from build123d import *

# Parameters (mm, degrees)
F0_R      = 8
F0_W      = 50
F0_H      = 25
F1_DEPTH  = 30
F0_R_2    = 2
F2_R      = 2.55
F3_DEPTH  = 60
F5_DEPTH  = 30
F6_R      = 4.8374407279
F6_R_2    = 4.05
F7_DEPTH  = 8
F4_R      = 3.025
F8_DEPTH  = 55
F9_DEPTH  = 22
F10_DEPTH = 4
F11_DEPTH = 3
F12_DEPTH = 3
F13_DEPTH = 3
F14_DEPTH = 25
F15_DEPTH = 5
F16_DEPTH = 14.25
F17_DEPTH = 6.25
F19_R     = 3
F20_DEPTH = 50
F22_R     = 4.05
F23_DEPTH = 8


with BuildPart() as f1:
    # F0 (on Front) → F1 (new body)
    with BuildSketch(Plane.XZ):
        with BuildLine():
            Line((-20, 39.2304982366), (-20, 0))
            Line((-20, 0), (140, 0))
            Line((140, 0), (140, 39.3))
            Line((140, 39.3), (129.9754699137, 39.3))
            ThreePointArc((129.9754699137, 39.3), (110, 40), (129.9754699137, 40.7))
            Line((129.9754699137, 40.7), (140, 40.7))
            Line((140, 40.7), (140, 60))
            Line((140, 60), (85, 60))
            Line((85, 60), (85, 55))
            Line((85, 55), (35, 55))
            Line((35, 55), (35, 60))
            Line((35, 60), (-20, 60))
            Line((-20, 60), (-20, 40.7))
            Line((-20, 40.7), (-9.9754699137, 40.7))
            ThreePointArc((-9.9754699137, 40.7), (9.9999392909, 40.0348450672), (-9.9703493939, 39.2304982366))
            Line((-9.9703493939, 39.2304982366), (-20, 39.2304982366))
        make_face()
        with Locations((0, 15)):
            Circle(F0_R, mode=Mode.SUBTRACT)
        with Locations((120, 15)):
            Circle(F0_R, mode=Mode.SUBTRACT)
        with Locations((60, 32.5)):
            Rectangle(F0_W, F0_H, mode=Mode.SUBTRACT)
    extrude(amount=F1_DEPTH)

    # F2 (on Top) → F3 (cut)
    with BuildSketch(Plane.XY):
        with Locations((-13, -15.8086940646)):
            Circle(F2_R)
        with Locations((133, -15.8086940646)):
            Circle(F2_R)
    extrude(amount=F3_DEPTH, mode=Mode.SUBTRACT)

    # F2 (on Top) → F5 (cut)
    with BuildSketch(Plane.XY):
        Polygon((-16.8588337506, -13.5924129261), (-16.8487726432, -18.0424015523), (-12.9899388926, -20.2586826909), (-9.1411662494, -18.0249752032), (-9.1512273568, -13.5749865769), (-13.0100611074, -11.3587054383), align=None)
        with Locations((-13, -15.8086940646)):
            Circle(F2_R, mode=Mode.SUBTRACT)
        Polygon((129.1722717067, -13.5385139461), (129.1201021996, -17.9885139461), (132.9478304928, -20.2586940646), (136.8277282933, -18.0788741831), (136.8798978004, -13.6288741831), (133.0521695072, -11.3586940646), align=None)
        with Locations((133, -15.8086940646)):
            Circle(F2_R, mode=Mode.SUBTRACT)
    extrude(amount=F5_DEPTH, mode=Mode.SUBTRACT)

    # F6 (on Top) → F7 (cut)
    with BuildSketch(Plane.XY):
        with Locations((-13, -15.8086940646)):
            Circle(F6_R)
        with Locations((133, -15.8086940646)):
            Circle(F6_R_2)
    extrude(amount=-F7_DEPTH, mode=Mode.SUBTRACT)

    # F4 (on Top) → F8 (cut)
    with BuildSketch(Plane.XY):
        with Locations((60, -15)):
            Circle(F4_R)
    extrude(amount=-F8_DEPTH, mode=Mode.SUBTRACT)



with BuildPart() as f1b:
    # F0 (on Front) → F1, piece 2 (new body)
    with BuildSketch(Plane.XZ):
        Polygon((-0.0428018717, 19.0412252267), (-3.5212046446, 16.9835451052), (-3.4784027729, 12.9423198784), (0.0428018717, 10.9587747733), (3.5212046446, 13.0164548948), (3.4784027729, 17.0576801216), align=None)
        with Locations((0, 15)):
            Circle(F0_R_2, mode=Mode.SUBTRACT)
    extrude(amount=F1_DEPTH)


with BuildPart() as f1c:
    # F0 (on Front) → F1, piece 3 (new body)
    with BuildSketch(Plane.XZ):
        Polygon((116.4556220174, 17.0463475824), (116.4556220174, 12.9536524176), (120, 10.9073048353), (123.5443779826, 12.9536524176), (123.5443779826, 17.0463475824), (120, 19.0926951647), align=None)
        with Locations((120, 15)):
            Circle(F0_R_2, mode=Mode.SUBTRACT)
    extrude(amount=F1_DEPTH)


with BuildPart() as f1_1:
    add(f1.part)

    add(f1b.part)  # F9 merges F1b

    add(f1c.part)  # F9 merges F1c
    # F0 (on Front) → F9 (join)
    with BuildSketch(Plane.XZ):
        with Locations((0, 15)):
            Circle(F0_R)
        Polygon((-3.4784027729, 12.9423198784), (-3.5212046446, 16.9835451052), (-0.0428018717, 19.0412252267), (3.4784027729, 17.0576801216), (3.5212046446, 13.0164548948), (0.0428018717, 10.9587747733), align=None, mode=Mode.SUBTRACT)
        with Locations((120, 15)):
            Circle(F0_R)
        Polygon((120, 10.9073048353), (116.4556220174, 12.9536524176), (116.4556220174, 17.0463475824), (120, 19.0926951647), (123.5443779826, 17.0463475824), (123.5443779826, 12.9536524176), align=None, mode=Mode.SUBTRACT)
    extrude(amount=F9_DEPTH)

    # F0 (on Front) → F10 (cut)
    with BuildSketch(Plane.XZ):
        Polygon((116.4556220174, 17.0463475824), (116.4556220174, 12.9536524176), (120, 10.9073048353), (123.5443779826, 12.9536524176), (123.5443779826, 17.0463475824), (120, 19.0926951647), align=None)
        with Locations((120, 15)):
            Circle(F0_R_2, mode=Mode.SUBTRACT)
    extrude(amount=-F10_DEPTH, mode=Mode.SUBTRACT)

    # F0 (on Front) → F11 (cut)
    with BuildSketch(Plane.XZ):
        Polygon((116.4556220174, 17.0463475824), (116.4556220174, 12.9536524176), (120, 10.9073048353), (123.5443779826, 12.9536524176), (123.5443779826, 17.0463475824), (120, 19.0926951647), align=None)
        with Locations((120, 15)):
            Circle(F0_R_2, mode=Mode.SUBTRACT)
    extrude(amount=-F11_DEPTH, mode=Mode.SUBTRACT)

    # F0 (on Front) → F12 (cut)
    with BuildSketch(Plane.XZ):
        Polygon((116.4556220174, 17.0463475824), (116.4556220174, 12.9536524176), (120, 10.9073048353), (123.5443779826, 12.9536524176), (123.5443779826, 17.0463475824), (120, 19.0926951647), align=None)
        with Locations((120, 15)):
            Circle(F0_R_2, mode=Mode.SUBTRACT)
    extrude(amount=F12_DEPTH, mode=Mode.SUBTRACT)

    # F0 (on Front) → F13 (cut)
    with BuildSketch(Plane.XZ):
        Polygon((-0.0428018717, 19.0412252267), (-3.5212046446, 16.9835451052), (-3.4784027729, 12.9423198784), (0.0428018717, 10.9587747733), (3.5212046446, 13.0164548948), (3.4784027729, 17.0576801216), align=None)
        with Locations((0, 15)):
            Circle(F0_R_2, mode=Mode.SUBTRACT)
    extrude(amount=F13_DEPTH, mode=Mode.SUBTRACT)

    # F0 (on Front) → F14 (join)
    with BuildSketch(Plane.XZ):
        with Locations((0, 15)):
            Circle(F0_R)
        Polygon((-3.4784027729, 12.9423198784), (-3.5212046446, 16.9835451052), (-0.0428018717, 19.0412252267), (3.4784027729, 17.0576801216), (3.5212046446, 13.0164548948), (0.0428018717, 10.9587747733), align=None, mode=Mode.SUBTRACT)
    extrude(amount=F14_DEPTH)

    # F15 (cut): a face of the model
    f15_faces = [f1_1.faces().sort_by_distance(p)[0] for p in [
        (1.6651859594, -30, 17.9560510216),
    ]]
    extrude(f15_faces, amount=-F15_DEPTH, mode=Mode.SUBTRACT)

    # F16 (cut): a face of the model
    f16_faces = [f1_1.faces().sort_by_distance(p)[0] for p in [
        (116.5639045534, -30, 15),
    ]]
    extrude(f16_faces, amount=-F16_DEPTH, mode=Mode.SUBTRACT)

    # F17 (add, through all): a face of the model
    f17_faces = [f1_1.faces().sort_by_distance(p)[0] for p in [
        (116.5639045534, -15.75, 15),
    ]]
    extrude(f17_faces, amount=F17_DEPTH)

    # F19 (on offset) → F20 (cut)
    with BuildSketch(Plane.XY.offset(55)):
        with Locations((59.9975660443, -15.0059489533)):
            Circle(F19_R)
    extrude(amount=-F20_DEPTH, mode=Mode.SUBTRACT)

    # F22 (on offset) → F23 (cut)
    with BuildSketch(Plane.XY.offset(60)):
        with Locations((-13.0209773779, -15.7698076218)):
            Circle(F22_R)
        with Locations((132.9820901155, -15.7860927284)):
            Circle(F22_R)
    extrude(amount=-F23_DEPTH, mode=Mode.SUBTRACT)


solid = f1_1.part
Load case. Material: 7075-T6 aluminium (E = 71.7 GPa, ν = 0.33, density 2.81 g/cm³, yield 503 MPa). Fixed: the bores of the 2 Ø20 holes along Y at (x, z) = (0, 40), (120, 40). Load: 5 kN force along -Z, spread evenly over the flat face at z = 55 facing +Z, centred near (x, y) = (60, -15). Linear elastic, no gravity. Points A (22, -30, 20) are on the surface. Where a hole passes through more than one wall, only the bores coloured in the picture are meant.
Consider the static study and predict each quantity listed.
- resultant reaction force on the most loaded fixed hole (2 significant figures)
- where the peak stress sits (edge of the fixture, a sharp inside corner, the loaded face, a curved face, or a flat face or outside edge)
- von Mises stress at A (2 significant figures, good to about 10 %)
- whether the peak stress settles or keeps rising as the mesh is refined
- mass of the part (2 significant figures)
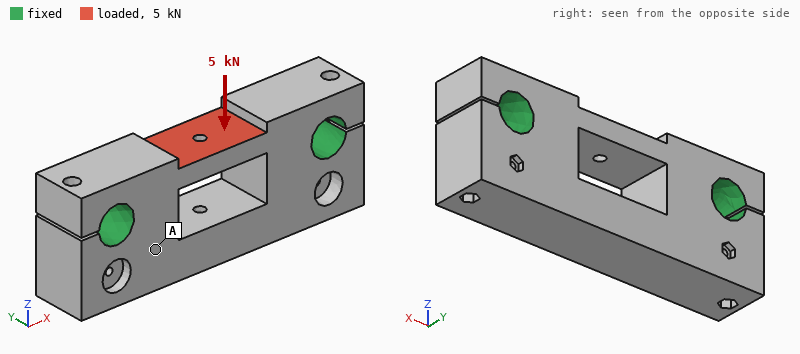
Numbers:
2.5 kN
a sharp inside corner
3.8 MPa
keeps rising
600 g
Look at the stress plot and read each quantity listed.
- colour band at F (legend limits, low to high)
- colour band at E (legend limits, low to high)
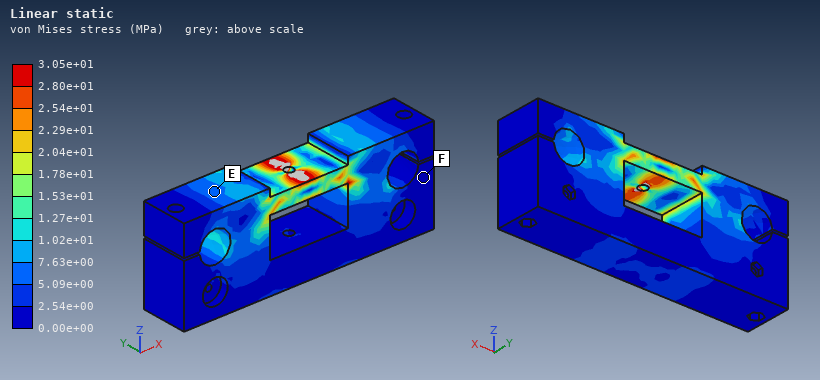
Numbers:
0.00e+00 to 2.54e+00 MPa
5.09e+00 to 7.63e+00 MPa
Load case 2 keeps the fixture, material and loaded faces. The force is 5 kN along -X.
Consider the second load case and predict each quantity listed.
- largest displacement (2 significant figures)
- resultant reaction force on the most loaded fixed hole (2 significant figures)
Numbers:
3.7 µm
2.5 kN
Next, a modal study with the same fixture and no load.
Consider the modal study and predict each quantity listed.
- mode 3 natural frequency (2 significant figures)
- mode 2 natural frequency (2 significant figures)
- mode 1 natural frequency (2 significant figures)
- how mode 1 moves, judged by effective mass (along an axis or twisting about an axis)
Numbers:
11 kHz
10 kHz
7800 Hz
along Y
